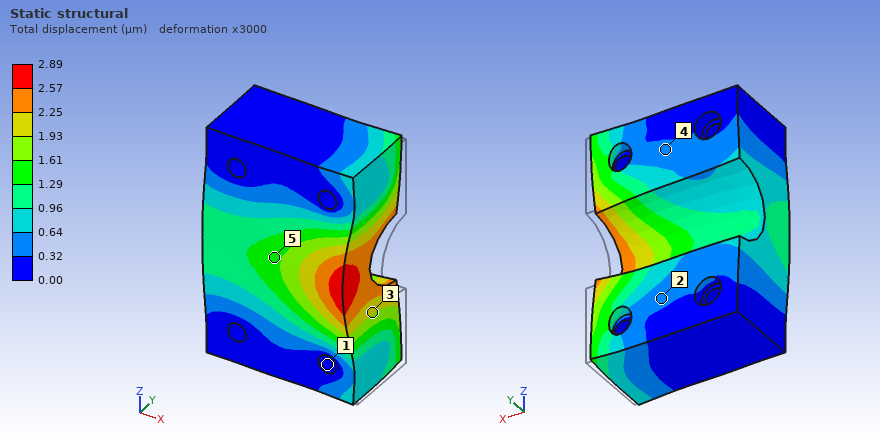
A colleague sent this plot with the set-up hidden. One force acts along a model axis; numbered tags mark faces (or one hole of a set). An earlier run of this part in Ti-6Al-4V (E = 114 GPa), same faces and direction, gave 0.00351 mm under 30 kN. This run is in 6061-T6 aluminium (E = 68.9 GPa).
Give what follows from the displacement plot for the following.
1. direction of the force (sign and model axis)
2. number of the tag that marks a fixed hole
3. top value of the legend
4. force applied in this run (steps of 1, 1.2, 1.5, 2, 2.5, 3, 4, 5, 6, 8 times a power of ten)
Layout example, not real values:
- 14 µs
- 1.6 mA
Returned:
- -X
- 1
- 2.89 µm
- 15 kN
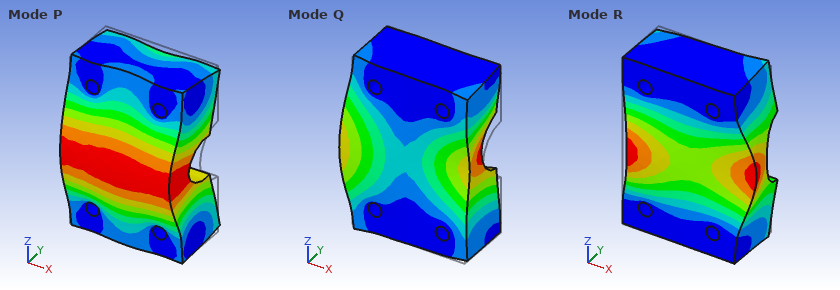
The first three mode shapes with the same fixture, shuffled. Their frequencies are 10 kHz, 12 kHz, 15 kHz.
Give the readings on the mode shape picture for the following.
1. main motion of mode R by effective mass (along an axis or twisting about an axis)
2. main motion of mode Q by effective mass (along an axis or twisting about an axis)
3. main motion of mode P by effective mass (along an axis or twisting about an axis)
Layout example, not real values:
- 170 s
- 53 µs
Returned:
- along X
- along X
- along Y
